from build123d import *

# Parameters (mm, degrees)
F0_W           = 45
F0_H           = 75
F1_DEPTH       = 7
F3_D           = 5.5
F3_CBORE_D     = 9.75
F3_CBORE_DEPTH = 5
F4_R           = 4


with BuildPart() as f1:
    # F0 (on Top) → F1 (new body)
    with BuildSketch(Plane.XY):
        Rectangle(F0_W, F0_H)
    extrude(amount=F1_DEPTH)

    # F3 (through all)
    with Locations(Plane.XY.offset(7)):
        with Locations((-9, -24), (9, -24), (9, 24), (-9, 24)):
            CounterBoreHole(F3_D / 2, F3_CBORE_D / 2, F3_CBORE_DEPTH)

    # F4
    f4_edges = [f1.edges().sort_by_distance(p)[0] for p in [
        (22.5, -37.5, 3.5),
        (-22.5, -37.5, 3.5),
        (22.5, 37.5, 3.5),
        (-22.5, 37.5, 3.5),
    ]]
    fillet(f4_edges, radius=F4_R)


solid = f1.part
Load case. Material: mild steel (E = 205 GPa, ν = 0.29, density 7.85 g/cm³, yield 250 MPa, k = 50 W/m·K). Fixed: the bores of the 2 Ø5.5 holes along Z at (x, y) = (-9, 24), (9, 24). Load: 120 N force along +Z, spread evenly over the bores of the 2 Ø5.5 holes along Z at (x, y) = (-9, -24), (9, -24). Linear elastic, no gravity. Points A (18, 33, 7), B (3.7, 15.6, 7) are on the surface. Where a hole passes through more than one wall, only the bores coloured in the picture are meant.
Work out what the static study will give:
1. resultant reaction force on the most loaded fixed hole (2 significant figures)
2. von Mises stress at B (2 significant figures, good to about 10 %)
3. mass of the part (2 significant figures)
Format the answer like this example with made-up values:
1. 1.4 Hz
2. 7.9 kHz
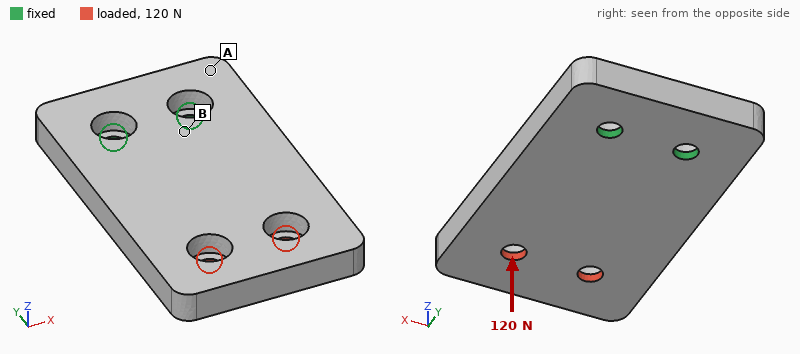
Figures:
1. 76 N
2. 17 MPa
3. 170 g
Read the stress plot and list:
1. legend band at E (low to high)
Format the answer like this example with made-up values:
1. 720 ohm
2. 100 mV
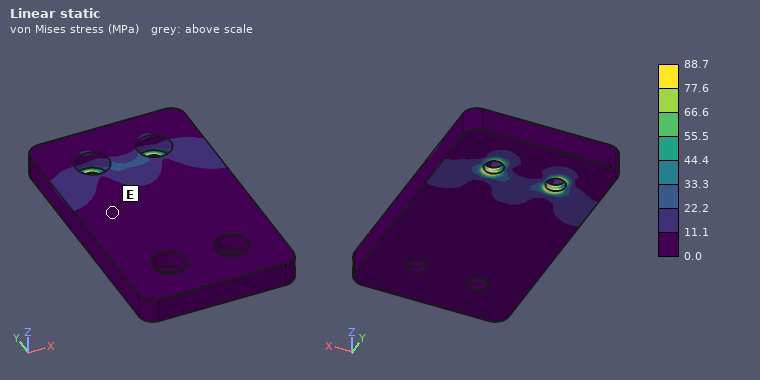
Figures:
1. 0.0 to 11.1 MPa
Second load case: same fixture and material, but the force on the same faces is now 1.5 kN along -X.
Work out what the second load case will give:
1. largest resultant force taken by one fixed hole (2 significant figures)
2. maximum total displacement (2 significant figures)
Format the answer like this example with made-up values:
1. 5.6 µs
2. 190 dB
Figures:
1. 3.4 kN
2. 37 µm
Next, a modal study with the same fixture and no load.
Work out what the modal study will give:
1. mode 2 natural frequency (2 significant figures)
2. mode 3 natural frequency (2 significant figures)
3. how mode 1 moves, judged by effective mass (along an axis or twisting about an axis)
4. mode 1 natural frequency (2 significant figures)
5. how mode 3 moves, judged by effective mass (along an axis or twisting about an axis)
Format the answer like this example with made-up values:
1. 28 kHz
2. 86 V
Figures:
1. 3800 Hz
2. 4500 Hz
3. along Z
4. 980 Hz
5. along X
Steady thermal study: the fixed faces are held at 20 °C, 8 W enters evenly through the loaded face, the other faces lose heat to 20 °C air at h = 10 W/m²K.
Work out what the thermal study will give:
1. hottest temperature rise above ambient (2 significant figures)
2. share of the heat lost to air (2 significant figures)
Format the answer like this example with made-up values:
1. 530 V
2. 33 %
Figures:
1. 32 K
2. 16 %
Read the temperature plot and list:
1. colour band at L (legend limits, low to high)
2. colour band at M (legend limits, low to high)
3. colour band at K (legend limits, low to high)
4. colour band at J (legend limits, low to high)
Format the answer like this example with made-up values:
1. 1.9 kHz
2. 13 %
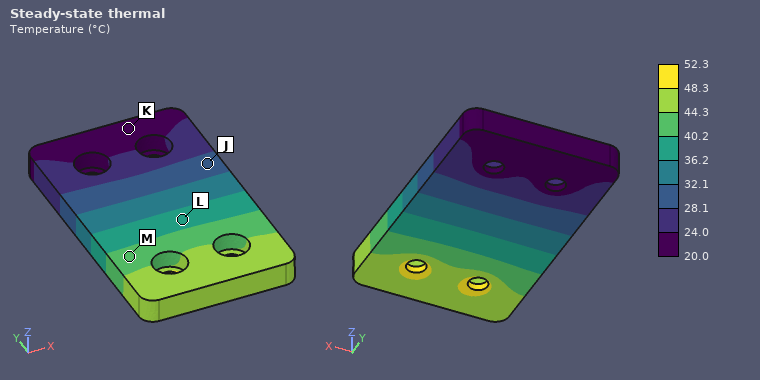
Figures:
1. 36.2 to 40.2 °C
2. 40.2 to 44.3 °C
3. 20.0 to 24.0 °C
4. 28.1 to 32.1 °C
